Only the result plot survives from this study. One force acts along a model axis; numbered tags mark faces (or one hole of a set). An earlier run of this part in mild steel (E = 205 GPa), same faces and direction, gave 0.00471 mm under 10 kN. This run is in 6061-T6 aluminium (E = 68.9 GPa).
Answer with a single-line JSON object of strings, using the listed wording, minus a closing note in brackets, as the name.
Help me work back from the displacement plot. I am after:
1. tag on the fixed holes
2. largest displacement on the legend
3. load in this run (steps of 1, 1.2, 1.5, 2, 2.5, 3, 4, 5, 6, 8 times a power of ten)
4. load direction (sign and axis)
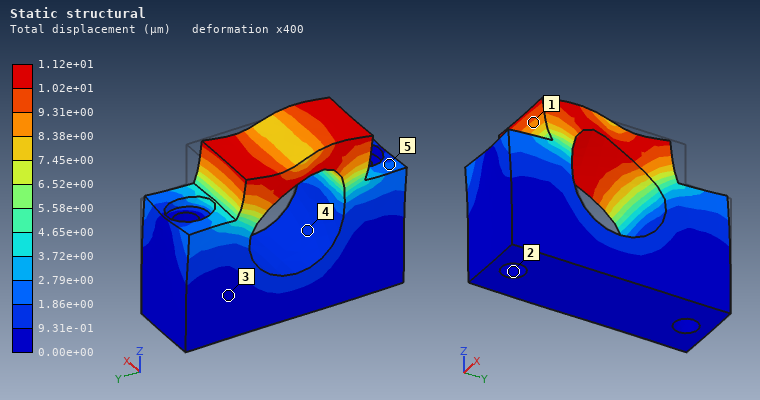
{"tag on the fixed holes": "2", "largest displacement on the legend": "1.12e+01 µm", "load in this run": "8 kN", "load direction": "-Y"}
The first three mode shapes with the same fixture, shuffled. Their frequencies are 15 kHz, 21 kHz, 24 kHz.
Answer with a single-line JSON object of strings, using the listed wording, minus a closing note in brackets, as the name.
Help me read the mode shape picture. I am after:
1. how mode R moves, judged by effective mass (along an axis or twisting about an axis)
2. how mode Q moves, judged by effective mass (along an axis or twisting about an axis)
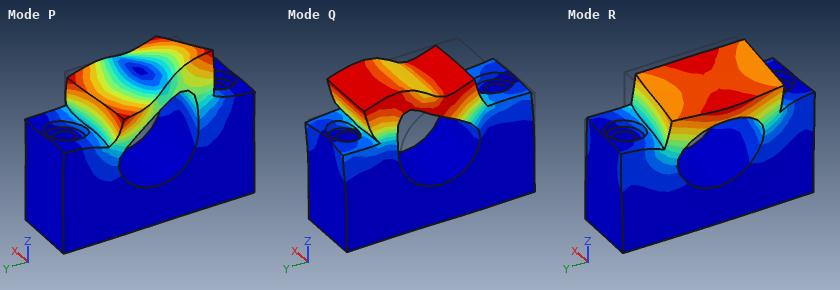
{"how mode R moves, judged by effective mass": "along X", "how mode Q moves, judged by effective mass": "along Y"}
